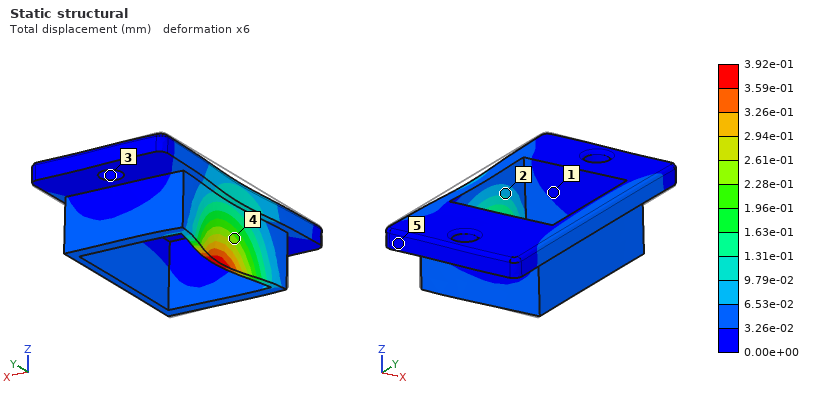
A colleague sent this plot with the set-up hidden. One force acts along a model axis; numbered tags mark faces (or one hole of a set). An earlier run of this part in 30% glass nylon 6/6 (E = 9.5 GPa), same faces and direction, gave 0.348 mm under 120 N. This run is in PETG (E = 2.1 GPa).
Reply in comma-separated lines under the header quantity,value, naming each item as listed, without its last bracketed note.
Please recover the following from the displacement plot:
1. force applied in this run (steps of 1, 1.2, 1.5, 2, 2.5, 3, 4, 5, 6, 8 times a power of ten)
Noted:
quantity,value
force applied in this run,30 N
